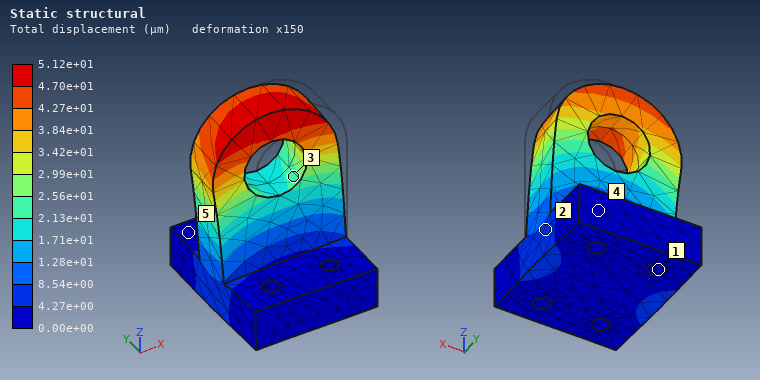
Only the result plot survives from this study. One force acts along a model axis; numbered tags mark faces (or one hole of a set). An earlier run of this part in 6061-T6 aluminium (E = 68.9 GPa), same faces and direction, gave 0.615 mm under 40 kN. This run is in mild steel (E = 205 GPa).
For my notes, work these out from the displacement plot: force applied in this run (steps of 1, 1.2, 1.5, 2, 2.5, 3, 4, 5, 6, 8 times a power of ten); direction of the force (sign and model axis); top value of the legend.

10 kN
-X
5.12e+01 µm
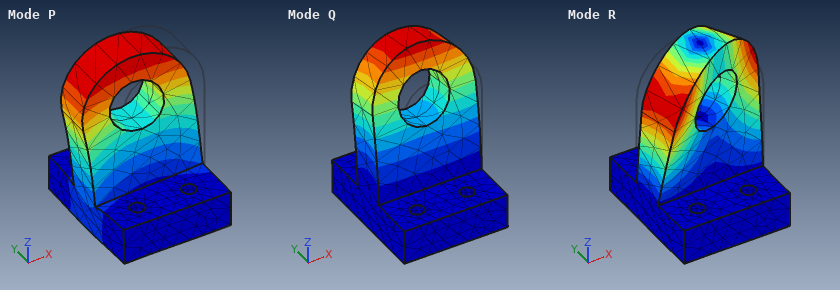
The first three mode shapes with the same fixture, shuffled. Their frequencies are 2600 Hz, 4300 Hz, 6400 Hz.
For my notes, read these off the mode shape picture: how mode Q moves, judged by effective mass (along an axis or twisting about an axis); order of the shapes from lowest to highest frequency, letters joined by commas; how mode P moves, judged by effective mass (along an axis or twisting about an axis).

along Y
Q, P, R
along X
